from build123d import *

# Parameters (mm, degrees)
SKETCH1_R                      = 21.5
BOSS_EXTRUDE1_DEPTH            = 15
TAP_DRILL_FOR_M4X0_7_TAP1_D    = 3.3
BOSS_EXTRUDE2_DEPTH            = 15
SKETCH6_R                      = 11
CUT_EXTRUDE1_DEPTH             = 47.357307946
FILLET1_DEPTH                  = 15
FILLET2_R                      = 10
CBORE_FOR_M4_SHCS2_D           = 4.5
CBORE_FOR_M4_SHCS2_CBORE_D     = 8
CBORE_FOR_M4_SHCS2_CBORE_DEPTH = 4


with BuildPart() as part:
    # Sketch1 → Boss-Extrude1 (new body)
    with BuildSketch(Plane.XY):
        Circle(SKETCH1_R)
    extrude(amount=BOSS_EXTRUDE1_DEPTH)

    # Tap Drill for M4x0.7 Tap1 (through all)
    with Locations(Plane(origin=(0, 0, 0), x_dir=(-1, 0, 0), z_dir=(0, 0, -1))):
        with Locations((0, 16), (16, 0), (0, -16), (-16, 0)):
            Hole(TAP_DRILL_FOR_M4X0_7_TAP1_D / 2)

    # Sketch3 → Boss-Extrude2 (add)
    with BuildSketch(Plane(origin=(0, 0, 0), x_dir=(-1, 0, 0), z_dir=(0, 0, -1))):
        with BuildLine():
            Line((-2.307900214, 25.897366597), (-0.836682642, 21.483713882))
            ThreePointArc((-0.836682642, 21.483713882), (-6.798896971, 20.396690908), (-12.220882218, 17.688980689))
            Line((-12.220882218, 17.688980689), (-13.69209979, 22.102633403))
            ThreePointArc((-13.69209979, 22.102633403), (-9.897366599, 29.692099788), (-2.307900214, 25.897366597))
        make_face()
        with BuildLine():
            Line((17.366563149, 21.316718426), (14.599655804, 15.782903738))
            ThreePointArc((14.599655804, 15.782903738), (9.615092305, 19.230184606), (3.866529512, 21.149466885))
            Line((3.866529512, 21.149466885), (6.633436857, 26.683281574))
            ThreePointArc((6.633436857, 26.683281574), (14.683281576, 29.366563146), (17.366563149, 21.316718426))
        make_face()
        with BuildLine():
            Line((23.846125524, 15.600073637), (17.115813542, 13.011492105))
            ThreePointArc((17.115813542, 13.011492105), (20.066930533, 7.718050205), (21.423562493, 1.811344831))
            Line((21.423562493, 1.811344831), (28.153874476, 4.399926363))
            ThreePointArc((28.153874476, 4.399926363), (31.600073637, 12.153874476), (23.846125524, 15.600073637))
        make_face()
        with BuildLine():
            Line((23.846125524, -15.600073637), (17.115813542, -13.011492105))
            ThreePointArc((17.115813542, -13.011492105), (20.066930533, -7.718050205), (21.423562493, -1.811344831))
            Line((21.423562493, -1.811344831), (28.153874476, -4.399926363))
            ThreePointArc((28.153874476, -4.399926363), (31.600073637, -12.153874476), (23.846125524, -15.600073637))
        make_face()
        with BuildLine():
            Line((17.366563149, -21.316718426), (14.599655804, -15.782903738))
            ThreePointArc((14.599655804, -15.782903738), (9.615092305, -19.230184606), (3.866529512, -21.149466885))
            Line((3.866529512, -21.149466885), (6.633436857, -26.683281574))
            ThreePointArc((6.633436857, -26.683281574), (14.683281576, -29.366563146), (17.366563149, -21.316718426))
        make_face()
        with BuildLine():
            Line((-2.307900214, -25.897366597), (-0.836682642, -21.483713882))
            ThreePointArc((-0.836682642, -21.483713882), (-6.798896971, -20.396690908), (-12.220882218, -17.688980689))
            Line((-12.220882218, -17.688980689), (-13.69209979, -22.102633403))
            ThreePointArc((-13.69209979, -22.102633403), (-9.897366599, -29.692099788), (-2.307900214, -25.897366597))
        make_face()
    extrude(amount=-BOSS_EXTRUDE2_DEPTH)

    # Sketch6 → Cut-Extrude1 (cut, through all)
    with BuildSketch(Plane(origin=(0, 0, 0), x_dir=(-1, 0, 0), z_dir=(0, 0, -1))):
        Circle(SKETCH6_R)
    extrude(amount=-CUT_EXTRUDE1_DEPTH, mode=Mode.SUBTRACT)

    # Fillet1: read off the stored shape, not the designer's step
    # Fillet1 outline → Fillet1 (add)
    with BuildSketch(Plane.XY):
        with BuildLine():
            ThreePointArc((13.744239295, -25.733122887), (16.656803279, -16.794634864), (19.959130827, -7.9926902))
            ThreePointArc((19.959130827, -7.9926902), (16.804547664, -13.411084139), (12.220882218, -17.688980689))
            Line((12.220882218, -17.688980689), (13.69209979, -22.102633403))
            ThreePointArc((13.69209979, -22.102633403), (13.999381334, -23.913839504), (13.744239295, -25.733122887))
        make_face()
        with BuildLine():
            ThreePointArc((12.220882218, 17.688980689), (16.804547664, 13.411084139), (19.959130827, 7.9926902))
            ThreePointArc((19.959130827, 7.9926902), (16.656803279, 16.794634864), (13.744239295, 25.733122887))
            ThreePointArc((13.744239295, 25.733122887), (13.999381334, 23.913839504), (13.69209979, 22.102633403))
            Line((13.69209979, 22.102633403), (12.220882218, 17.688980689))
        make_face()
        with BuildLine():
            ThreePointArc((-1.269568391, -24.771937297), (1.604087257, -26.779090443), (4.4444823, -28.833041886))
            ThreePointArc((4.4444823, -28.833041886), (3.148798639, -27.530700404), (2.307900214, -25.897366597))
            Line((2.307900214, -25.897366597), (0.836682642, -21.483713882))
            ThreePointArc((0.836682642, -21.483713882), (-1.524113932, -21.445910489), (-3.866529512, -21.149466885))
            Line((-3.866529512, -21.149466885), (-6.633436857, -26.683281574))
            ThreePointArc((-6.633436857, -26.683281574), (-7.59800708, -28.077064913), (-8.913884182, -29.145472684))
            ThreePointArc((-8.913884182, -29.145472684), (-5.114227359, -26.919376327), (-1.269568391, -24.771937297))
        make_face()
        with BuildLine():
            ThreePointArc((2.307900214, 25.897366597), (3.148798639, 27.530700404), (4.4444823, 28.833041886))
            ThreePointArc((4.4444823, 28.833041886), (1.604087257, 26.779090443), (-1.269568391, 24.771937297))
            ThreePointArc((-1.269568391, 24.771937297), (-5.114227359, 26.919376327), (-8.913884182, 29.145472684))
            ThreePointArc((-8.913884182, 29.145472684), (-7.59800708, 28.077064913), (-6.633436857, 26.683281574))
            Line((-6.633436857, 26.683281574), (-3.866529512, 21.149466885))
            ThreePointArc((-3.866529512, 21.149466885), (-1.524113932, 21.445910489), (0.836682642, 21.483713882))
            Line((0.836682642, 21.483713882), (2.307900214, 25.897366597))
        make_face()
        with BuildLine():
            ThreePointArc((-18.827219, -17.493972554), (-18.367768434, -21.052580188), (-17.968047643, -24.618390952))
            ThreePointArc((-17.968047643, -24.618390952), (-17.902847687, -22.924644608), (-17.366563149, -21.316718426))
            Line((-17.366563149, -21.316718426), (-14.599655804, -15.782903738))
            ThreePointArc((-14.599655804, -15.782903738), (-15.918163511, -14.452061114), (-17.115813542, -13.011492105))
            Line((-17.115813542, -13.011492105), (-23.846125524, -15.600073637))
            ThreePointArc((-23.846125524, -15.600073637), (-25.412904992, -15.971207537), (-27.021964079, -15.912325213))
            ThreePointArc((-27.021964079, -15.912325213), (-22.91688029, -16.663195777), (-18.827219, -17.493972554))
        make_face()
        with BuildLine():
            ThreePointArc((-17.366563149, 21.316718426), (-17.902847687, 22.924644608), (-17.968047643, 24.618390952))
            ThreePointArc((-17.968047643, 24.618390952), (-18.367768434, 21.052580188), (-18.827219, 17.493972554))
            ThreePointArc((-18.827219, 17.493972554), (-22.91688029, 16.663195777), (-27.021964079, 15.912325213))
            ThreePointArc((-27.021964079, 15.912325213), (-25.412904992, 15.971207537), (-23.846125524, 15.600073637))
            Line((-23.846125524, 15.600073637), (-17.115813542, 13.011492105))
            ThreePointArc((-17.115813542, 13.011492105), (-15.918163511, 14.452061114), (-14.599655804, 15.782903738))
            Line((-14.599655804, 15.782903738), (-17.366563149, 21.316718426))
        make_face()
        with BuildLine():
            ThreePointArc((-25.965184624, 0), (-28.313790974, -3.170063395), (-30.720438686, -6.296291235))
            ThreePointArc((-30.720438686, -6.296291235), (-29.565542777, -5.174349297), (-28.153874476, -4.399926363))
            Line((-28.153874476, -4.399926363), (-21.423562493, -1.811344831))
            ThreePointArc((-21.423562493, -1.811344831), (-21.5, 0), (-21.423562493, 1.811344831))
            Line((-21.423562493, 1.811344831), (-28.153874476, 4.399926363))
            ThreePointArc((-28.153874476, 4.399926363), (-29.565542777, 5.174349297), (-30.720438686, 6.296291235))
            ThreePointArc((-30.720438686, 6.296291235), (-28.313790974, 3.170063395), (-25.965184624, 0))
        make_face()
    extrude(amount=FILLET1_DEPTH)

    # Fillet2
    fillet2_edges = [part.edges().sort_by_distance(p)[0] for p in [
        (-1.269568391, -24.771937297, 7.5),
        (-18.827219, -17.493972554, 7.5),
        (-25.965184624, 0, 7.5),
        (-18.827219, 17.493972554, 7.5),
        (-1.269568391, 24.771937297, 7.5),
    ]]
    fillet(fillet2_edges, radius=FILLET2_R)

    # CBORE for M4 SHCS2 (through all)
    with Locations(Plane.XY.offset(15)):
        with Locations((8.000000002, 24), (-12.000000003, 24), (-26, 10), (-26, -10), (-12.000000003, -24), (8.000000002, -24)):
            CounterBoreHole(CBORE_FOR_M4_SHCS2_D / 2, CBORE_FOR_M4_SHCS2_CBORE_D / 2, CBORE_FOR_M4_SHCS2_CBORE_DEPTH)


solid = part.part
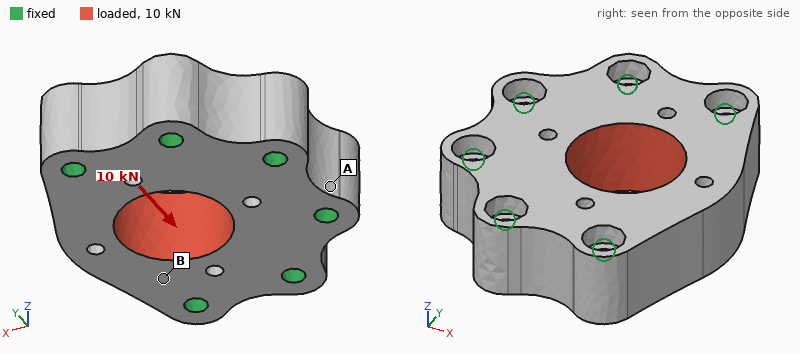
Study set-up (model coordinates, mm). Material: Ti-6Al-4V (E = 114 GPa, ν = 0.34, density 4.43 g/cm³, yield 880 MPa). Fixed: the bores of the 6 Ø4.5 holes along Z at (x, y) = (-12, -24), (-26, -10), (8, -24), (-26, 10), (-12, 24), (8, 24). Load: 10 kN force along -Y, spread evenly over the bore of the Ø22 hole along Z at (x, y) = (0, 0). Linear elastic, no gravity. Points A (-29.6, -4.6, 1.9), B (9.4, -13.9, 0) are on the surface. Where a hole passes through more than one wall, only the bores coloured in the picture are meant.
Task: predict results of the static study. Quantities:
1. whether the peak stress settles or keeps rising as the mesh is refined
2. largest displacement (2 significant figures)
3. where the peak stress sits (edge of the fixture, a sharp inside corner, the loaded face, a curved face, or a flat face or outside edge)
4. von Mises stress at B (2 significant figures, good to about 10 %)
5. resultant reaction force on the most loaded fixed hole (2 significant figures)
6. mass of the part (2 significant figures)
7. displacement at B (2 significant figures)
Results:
keeps rising
2.9 µm
edge of the fixture
16 MPa
2.8 kN
130 g
1.4 µm
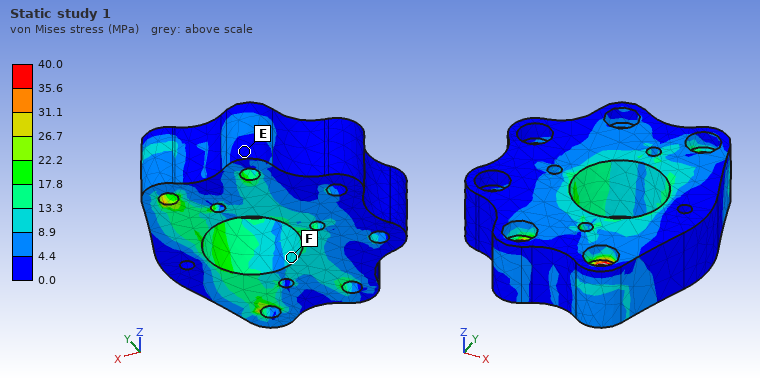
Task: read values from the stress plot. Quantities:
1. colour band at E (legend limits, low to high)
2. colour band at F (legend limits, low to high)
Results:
0.0 to 4.4 MPa
8.9 to 13.3 MPa
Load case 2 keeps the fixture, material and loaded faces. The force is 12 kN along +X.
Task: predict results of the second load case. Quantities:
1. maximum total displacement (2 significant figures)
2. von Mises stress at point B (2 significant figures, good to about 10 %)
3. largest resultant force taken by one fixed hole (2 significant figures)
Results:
8.4 µm
15 MPa
2.6 kN
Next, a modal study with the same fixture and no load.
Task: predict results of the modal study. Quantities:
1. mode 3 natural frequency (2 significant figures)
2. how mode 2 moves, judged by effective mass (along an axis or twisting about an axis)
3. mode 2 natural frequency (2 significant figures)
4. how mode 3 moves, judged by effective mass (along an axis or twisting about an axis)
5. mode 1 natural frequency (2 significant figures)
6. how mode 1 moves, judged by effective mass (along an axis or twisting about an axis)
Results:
33 kHz
along X
31 kHz
along Z
18 kHz
along Z
